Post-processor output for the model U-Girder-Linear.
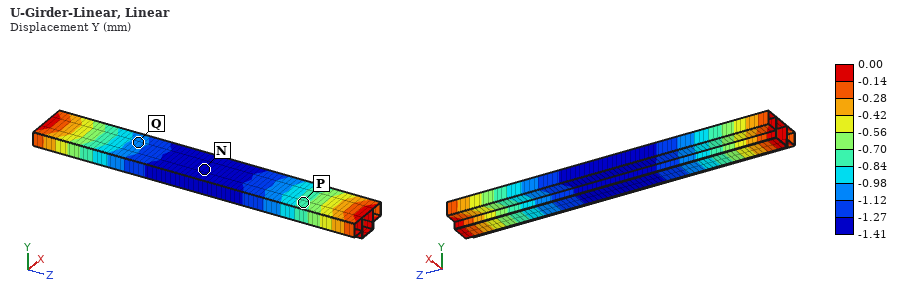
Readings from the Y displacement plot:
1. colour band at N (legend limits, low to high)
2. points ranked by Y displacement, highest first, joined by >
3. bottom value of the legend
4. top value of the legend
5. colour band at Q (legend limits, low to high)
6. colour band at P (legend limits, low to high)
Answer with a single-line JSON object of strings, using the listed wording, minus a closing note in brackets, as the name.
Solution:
{"colour band at N": "-1.41 to -1.27 mm", "points ranked by Y displacement, highest first, joined by >": "P > Q > N", "bottom value of the legend": "-1.41 mm", "top value of the legend": "0.00 mm", "colour band at Q": "-1.12 to -0.98 mm", "colour band at P": "-0.84 to -0.70 mm"}
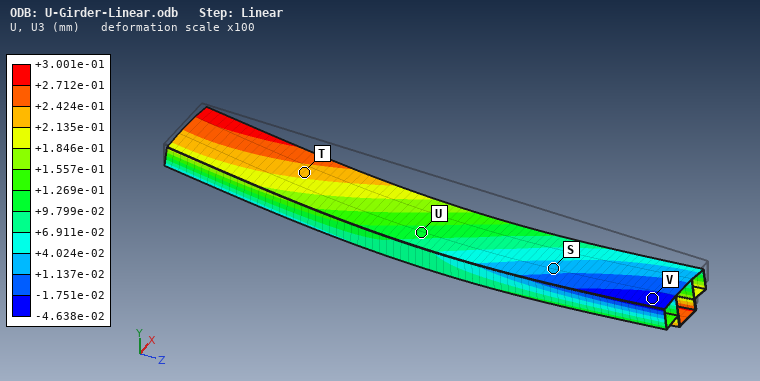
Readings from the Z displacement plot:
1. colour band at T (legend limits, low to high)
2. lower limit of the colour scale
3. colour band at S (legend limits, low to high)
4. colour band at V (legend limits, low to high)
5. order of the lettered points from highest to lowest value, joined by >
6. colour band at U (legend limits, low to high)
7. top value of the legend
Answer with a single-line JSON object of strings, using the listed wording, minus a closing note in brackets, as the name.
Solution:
{"colour band at T": "+2.135e-01 to +2.424e-01 mm", "lower limit of the colour scale": "-4.638e-02 mm", "colour band at S": "+1.137e-02 to +4.024e-02 mm", "colour band at V": "-4.638e-02 to -1.751e-02 mm", "order of the lettered points from highest to lowest value, joined by >": "T > U > S > V", "colour band at U": "+9.799e-02 to +1.269e-01 mm", "top value of the legend": "+3.001e-01 mm"}
